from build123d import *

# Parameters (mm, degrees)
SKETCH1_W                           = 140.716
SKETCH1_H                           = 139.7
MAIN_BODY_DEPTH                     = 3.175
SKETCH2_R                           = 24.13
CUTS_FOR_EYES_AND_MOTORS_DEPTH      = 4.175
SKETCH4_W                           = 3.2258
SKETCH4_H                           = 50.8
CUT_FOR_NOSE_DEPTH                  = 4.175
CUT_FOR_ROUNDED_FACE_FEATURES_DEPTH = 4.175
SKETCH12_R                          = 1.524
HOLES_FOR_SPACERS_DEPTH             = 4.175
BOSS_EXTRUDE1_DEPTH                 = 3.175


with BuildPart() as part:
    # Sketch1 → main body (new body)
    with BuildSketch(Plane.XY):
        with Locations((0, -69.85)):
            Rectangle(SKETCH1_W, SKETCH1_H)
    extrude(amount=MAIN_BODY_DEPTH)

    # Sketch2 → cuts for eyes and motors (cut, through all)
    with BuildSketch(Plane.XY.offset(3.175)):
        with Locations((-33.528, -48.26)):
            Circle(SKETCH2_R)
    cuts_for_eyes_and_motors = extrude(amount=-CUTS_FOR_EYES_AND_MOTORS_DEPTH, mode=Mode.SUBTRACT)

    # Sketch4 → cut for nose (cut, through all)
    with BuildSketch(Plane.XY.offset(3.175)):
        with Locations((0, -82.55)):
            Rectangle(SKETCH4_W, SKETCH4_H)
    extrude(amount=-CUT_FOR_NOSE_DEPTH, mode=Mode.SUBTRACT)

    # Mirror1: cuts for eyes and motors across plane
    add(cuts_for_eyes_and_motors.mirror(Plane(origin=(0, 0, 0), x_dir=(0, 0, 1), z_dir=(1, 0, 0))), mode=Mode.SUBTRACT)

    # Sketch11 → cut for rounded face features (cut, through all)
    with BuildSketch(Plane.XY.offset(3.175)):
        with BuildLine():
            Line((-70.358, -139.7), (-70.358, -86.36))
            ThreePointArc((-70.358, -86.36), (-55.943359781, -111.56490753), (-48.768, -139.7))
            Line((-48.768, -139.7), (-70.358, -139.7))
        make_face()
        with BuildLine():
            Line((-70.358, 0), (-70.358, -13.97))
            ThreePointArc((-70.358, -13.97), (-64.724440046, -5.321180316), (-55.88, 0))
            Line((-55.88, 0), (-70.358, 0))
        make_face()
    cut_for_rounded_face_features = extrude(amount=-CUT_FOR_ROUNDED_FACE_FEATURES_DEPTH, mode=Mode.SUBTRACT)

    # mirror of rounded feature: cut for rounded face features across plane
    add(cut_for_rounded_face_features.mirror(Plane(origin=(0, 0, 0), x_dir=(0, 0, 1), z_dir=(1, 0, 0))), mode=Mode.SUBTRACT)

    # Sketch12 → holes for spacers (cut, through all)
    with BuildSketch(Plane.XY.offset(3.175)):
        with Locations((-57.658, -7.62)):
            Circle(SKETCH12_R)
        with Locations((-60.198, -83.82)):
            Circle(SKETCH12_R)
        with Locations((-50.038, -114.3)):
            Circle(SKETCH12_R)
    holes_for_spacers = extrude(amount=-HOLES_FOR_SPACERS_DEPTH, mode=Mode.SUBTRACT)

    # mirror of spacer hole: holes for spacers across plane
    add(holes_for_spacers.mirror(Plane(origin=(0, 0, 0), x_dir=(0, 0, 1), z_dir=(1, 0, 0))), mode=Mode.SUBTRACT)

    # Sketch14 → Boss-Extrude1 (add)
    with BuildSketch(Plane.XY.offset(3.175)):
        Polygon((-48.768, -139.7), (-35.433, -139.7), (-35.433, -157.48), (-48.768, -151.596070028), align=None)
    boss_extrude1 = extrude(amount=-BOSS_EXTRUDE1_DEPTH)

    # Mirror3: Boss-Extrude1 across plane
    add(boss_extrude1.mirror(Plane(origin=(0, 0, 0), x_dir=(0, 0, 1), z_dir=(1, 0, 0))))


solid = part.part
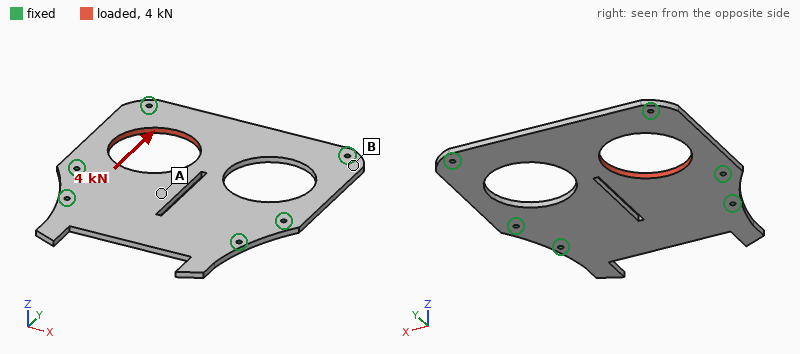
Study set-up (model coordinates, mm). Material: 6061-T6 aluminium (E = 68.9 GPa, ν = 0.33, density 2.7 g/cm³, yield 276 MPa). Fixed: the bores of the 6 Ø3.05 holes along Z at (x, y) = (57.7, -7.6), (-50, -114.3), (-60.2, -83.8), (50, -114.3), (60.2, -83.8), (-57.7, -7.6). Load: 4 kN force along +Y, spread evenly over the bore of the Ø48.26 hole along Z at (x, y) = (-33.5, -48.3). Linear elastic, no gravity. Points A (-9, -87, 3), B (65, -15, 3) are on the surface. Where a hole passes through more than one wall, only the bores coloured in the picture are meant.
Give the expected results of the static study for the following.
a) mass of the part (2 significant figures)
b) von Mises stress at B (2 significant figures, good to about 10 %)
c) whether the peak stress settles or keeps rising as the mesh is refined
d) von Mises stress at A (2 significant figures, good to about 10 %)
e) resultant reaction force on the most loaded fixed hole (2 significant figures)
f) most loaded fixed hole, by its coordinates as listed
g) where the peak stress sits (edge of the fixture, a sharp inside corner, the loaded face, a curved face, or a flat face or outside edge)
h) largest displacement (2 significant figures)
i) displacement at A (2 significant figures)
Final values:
130 g
2.7 MPa
keeps rising
9.2 MPa
1.3 kN
(-57.7, -7.6)
edge of the fixture
23 µm
14 µm
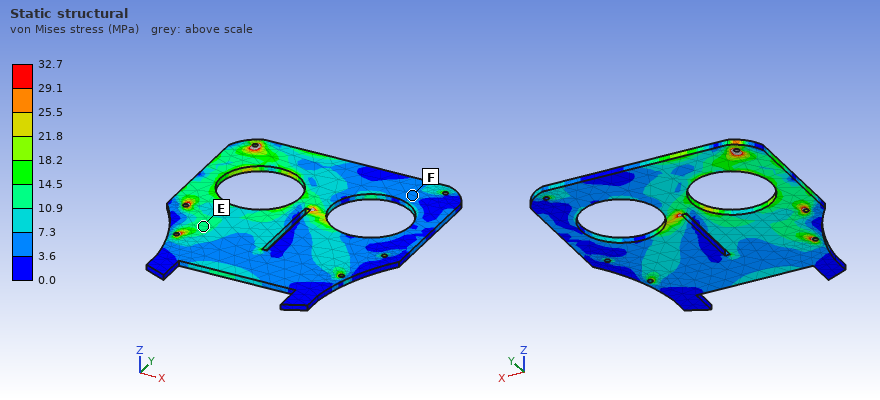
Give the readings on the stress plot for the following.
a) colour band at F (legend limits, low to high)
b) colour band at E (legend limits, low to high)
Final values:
3.6 to 7.3 MPa
10.9 to 14.5 MPa
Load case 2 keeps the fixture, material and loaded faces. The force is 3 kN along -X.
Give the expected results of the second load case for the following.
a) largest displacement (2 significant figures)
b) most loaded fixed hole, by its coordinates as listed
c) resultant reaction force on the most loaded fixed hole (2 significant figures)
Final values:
22 µm
(-60.2, -83.8)
1.1 kN
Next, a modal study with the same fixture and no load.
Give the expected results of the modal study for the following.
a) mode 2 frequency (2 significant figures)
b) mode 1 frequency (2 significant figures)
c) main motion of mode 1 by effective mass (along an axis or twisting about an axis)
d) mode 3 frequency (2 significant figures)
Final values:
1300 Hz
1000 Hz
along Z
1500 Hz
